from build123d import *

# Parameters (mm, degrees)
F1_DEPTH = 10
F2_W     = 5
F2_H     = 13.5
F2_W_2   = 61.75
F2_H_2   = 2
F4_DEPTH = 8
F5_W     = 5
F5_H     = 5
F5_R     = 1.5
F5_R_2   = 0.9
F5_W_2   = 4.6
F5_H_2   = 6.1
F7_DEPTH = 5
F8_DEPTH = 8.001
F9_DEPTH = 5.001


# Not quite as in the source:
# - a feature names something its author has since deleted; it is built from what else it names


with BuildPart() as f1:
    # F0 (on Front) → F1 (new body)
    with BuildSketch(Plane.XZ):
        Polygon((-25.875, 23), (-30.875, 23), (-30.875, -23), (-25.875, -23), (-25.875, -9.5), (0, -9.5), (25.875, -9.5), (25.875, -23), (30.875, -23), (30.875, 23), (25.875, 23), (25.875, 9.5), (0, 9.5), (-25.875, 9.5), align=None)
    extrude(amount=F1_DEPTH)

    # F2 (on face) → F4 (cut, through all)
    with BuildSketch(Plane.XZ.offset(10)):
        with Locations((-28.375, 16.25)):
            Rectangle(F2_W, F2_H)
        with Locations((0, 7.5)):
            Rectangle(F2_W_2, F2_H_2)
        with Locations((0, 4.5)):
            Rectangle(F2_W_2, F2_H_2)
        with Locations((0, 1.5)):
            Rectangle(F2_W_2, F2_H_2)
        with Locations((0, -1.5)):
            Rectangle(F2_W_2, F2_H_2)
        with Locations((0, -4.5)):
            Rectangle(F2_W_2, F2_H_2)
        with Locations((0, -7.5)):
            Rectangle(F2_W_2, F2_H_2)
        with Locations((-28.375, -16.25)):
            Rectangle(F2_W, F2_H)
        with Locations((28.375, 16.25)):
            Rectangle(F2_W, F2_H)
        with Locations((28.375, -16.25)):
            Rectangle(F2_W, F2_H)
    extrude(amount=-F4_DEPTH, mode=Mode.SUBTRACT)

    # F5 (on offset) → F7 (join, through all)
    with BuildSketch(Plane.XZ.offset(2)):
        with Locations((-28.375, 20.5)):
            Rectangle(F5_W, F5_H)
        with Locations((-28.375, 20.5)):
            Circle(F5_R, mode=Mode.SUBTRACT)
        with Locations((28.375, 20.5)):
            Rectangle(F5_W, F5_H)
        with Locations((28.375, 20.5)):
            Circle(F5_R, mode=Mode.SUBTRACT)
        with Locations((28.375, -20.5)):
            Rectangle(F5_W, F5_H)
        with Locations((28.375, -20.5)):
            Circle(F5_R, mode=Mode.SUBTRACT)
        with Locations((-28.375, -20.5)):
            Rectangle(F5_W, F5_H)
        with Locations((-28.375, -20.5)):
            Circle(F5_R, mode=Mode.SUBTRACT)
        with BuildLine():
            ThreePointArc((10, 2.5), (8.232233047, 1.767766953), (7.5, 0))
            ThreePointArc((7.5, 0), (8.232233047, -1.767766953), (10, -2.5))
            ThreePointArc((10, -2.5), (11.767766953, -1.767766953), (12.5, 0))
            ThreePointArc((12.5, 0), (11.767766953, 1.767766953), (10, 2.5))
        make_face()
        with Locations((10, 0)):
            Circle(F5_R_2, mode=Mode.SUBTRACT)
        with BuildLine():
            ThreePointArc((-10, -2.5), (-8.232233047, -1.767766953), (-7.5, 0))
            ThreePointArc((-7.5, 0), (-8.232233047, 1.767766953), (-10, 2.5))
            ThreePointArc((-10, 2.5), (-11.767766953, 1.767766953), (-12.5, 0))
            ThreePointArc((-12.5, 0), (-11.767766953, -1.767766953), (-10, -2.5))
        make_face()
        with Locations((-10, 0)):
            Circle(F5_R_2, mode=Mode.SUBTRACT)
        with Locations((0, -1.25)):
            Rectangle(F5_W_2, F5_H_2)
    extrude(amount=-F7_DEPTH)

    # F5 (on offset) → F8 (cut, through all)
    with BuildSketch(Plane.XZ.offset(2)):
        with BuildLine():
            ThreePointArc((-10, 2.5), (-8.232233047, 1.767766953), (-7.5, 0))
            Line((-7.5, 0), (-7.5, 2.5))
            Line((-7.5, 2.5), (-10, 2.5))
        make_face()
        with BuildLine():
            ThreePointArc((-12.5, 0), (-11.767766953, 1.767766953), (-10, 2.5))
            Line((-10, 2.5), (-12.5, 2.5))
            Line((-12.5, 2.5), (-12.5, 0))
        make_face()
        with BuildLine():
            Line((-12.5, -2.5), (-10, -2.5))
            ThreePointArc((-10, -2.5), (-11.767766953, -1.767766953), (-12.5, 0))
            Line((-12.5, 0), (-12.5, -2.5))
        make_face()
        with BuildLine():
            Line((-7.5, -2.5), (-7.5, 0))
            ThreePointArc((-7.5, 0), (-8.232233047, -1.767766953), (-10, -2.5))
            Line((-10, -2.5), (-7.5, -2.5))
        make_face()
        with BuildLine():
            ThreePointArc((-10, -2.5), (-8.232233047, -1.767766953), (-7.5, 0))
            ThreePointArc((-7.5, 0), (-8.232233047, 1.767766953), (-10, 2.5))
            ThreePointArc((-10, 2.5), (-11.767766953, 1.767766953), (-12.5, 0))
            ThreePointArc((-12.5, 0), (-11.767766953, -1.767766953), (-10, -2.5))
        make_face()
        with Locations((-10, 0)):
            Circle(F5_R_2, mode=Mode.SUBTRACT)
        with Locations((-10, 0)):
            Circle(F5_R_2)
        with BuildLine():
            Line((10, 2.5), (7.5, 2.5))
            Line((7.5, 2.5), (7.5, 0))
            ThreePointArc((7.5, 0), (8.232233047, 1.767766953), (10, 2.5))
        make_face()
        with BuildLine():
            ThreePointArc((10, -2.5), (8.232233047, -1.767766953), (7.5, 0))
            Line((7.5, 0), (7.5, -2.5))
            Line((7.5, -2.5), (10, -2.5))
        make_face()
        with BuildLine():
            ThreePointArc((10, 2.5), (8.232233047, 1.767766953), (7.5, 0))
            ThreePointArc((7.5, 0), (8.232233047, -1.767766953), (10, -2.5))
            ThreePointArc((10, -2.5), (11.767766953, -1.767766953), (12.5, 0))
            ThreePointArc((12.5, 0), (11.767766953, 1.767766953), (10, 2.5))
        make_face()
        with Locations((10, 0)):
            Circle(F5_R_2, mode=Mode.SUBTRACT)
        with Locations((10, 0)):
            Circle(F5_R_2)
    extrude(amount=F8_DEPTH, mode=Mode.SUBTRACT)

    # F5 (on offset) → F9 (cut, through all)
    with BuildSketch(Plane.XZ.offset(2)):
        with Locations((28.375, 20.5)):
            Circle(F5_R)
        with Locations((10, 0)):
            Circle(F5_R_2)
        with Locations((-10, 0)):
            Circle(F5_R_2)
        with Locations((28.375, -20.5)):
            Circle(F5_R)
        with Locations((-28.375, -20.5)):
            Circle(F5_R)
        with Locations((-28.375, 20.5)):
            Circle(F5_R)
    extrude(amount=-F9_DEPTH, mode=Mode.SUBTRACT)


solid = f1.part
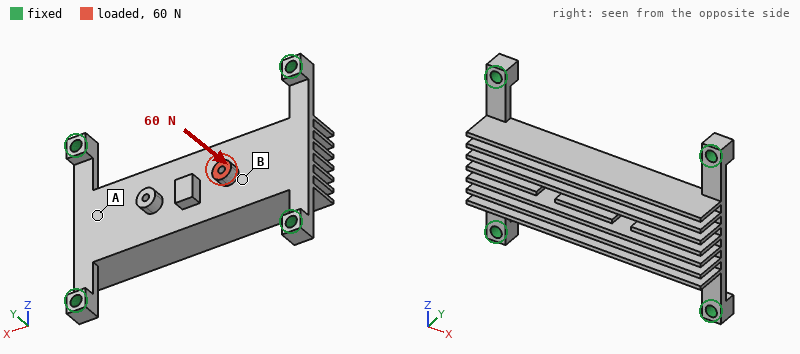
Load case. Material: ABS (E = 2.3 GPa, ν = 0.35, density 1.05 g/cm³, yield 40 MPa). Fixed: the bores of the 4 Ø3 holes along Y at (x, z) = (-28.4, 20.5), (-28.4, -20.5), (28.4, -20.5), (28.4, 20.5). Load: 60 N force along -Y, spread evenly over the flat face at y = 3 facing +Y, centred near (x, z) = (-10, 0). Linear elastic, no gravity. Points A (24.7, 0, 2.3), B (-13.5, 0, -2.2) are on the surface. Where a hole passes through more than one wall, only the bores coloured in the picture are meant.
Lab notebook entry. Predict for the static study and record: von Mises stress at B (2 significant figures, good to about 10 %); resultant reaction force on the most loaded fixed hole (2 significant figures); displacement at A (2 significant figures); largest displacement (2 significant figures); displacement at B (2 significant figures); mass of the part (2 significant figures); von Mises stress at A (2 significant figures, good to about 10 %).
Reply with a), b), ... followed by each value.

a) 7.6 MPa
b) 22 N
c) 0.30 mm
d) 0.65 mm
e) 0.60 mm
f) 6.9 g
g) 3.5 MPa
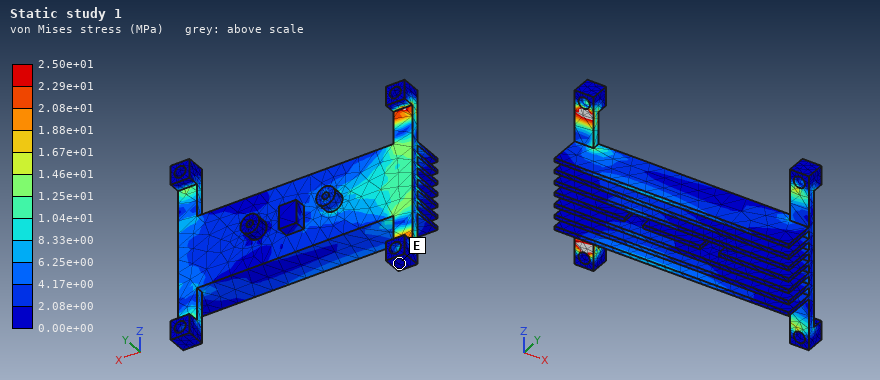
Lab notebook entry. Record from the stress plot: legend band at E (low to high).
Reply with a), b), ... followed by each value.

a) 0.00e+00 to 2.08e+00 MPa
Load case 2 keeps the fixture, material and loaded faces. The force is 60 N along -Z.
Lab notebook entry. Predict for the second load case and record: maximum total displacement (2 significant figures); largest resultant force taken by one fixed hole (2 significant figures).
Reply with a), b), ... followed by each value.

a) 0.16 mm
b) 22 N
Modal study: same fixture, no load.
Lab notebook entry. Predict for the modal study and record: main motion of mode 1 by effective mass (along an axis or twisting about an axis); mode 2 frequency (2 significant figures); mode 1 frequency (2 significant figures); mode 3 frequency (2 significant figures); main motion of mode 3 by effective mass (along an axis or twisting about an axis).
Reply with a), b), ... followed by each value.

a) along Y
b) 1200 Hz
c) 750 Hz
d) 1300 Hz
e) along Z
